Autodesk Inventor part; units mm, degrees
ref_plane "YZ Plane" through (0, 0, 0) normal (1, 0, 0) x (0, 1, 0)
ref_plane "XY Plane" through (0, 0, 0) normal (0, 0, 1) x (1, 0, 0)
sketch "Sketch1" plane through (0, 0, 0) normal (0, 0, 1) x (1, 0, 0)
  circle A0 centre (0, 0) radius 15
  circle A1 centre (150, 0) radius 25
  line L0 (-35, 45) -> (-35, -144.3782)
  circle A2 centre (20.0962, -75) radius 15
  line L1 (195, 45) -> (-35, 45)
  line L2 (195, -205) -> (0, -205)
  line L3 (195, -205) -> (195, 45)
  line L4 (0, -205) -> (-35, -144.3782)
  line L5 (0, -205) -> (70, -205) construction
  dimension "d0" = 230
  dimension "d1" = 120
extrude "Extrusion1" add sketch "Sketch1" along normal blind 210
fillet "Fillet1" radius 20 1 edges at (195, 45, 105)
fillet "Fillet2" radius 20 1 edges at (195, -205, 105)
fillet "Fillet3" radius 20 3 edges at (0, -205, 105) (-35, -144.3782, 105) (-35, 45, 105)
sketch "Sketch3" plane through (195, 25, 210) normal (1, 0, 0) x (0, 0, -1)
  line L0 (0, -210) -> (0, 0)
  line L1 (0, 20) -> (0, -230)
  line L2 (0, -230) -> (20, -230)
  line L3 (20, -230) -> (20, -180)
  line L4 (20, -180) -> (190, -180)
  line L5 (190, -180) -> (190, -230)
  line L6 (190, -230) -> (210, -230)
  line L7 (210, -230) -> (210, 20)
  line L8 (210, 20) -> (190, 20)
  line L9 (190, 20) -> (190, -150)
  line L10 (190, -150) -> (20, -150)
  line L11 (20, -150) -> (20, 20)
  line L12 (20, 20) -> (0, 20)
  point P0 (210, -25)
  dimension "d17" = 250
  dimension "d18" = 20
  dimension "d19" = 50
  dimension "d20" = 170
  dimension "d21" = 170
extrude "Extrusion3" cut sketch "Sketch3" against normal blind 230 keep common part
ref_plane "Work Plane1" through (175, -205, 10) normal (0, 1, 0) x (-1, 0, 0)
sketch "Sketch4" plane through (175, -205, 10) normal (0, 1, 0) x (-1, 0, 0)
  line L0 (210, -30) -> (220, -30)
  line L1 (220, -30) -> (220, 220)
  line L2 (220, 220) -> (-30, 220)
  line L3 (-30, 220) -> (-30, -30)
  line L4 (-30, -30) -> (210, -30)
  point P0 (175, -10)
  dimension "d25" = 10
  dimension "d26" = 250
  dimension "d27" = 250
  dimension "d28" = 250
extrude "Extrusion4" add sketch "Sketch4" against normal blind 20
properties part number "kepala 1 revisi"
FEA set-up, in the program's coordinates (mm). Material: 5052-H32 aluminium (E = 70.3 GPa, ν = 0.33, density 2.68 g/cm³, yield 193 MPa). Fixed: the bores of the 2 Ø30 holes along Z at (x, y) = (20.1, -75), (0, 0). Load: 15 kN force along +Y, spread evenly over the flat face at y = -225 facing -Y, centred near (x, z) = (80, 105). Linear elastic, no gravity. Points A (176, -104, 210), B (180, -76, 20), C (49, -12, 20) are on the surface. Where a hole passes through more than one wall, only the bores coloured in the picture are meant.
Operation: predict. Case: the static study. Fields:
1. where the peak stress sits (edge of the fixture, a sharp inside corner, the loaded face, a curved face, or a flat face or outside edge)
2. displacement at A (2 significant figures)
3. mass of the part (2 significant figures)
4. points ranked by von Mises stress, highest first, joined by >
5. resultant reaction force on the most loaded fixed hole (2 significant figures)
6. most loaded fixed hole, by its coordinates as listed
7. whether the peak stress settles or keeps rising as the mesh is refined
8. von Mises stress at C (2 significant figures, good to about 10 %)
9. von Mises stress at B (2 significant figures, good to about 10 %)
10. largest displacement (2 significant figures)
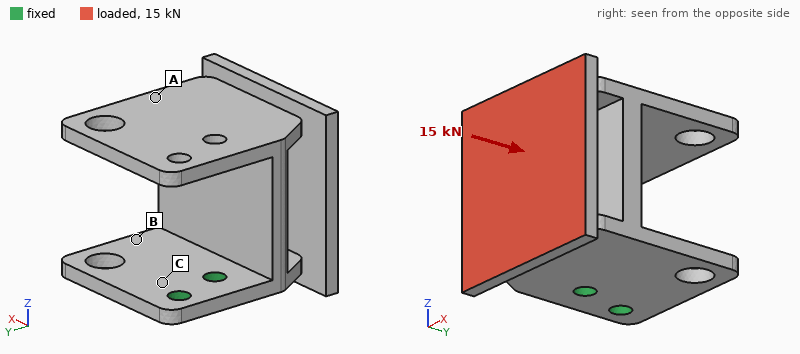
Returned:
edge of the fixture
2.1 mm
12 kg
B > C > A
17 kN
(20.1, -75)
keeps rising
23 MPa
46 MPa
2.7 mm
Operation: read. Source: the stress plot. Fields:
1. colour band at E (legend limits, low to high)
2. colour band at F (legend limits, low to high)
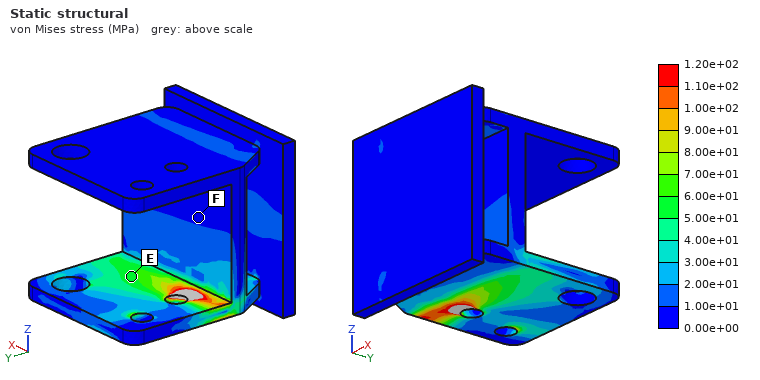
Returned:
5.00e+01 to 6.00e+01 MPa
0.00e+00 to 1.00e+01 MPa
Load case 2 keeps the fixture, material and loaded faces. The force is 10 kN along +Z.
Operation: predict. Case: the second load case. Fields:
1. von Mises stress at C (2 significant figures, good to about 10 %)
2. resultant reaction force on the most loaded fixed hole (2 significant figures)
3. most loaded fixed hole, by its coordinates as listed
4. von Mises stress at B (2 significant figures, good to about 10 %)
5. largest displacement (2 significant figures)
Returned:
17 MPa
16 kN
(20.1, -75)
34 MPa
2.6 mm
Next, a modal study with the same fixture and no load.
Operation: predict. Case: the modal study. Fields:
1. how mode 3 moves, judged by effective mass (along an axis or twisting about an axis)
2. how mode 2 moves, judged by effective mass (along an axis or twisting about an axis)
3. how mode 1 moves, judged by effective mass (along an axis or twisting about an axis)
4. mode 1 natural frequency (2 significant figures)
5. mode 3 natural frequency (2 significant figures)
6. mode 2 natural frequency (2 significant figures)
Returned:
along Z
along X
along Y
110 Hz
480 Hz
170 Hz
